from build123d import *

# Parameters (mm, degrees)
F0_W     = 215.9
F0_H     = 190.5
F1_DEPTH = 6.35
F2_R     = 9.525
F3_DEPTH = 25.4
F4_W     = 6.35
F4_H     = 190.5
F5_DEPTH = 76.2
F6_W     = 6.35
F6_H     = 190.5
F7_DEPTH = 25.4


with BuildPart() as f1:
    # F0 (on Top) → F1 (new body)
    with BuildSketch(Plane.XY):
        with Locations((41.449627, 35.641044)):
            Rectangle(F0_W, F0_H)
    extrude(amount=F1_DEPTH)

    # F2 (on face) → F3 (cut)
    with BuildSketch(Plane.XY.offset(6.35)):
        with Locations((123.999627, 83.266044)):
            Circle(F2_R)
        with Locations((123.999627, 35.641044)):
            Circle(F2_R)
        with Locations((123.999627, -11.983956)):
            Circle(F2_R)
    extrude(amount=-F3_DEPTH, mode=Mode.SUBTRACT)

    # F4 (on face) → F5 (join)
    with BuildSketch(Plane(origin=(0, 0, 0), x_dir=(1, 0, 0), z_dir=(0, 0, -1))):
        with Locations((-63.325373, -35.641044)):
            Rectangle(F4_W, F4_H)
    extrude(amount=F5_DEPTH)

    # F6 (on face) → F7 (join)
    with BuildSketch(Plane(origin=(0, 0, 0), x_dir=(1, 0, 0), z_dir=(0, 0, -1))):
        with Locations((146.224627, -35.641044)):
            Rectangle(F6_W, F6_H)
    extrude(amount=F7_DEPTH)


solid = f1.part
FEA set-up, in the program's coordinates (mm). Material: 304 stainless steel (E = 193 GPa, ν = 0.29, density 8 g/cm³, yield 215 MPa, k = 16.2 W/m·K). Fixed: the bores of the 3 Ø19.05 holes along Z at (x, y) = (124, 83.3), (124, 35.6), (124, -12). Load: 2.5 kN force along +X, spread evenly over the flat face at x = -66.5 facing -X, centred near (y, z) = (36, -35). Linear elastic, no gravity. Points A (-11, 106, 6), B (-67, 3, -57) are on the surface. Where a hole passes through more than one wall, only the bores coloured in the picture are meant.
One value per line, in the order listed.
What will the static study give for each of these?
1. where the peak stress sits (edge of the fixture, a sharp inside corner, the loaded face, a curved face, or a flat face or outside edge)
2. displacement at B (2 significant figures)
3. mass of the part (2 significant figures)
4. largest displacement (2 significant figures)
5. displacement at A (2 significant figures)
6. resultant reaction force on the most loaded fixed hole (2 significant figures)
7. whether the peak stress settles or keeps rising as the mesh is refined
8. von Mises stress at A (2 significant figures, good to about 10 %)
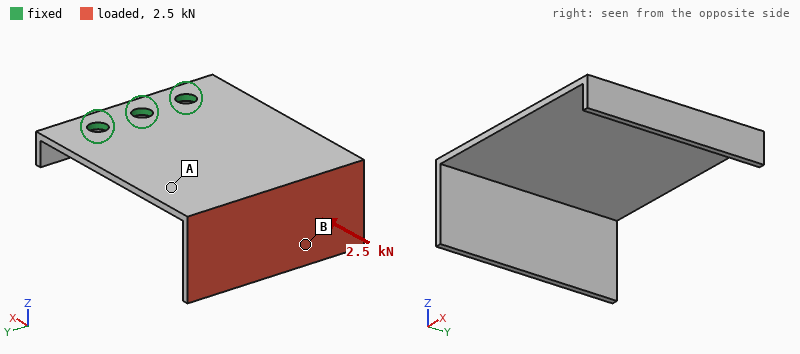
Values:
edge of the fixture
2.4 mm
3.0 kg
2.7 mm
0.96 mm
970 N
keeps rising
70 MPa
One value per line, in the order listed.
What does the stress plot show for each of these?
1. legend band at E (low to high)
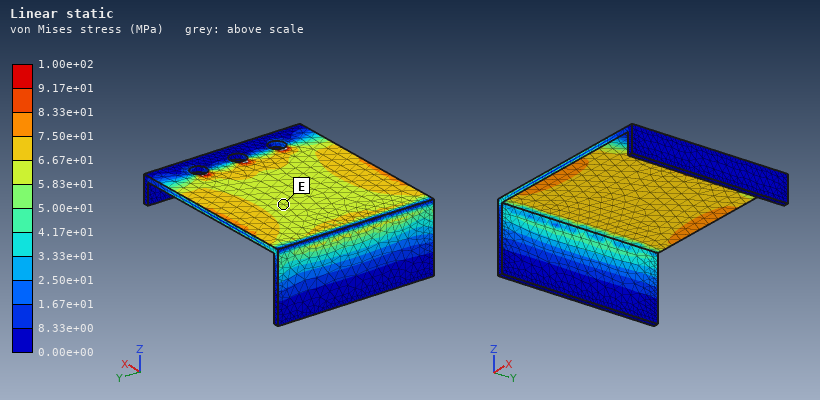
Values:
5.83e+01 to 6.67e+01 MPa
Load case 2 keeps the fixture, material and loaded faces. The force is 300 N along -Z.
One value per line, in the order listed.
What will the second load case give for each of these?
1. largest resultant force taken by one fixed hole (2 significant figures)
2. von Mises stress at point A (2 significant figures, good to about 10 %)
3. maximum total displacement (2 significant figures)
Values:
200 N
13 MPa
0.91 mm
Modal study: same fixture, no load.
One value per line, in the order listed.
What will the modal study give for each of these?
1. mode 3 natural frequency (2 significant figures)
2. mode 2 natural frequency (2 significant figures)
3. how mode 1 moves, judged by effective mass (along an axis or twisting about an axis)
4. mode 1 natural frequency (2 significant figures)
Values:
410 Hz
210 Hz
along Z
90 Hz
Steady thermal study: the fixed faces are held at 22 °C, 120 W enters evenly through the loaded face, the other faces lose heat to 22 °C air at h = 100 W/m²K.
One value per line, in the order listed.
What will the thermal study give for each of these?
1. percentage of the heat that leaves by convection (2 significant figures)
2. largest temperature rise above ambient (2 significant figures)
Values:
100 %
64 K
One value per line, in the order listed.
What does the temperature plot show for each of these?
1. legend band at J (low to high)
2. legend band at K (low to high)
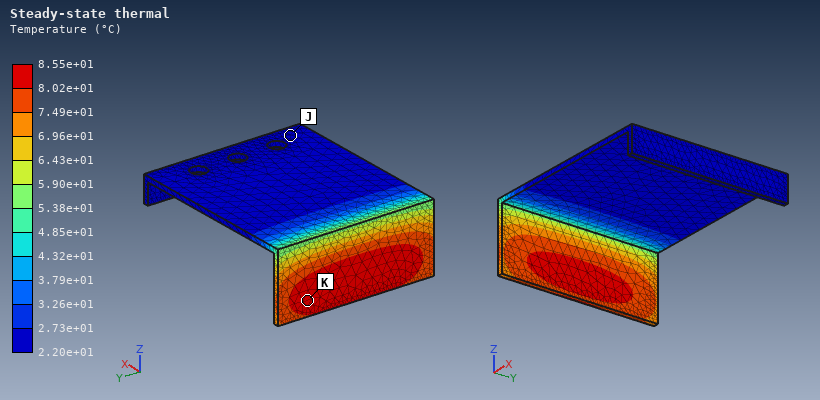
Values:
2.20e+01 to 2.73e+01 °C
8.02e+01 to 8.55e+01 °C
